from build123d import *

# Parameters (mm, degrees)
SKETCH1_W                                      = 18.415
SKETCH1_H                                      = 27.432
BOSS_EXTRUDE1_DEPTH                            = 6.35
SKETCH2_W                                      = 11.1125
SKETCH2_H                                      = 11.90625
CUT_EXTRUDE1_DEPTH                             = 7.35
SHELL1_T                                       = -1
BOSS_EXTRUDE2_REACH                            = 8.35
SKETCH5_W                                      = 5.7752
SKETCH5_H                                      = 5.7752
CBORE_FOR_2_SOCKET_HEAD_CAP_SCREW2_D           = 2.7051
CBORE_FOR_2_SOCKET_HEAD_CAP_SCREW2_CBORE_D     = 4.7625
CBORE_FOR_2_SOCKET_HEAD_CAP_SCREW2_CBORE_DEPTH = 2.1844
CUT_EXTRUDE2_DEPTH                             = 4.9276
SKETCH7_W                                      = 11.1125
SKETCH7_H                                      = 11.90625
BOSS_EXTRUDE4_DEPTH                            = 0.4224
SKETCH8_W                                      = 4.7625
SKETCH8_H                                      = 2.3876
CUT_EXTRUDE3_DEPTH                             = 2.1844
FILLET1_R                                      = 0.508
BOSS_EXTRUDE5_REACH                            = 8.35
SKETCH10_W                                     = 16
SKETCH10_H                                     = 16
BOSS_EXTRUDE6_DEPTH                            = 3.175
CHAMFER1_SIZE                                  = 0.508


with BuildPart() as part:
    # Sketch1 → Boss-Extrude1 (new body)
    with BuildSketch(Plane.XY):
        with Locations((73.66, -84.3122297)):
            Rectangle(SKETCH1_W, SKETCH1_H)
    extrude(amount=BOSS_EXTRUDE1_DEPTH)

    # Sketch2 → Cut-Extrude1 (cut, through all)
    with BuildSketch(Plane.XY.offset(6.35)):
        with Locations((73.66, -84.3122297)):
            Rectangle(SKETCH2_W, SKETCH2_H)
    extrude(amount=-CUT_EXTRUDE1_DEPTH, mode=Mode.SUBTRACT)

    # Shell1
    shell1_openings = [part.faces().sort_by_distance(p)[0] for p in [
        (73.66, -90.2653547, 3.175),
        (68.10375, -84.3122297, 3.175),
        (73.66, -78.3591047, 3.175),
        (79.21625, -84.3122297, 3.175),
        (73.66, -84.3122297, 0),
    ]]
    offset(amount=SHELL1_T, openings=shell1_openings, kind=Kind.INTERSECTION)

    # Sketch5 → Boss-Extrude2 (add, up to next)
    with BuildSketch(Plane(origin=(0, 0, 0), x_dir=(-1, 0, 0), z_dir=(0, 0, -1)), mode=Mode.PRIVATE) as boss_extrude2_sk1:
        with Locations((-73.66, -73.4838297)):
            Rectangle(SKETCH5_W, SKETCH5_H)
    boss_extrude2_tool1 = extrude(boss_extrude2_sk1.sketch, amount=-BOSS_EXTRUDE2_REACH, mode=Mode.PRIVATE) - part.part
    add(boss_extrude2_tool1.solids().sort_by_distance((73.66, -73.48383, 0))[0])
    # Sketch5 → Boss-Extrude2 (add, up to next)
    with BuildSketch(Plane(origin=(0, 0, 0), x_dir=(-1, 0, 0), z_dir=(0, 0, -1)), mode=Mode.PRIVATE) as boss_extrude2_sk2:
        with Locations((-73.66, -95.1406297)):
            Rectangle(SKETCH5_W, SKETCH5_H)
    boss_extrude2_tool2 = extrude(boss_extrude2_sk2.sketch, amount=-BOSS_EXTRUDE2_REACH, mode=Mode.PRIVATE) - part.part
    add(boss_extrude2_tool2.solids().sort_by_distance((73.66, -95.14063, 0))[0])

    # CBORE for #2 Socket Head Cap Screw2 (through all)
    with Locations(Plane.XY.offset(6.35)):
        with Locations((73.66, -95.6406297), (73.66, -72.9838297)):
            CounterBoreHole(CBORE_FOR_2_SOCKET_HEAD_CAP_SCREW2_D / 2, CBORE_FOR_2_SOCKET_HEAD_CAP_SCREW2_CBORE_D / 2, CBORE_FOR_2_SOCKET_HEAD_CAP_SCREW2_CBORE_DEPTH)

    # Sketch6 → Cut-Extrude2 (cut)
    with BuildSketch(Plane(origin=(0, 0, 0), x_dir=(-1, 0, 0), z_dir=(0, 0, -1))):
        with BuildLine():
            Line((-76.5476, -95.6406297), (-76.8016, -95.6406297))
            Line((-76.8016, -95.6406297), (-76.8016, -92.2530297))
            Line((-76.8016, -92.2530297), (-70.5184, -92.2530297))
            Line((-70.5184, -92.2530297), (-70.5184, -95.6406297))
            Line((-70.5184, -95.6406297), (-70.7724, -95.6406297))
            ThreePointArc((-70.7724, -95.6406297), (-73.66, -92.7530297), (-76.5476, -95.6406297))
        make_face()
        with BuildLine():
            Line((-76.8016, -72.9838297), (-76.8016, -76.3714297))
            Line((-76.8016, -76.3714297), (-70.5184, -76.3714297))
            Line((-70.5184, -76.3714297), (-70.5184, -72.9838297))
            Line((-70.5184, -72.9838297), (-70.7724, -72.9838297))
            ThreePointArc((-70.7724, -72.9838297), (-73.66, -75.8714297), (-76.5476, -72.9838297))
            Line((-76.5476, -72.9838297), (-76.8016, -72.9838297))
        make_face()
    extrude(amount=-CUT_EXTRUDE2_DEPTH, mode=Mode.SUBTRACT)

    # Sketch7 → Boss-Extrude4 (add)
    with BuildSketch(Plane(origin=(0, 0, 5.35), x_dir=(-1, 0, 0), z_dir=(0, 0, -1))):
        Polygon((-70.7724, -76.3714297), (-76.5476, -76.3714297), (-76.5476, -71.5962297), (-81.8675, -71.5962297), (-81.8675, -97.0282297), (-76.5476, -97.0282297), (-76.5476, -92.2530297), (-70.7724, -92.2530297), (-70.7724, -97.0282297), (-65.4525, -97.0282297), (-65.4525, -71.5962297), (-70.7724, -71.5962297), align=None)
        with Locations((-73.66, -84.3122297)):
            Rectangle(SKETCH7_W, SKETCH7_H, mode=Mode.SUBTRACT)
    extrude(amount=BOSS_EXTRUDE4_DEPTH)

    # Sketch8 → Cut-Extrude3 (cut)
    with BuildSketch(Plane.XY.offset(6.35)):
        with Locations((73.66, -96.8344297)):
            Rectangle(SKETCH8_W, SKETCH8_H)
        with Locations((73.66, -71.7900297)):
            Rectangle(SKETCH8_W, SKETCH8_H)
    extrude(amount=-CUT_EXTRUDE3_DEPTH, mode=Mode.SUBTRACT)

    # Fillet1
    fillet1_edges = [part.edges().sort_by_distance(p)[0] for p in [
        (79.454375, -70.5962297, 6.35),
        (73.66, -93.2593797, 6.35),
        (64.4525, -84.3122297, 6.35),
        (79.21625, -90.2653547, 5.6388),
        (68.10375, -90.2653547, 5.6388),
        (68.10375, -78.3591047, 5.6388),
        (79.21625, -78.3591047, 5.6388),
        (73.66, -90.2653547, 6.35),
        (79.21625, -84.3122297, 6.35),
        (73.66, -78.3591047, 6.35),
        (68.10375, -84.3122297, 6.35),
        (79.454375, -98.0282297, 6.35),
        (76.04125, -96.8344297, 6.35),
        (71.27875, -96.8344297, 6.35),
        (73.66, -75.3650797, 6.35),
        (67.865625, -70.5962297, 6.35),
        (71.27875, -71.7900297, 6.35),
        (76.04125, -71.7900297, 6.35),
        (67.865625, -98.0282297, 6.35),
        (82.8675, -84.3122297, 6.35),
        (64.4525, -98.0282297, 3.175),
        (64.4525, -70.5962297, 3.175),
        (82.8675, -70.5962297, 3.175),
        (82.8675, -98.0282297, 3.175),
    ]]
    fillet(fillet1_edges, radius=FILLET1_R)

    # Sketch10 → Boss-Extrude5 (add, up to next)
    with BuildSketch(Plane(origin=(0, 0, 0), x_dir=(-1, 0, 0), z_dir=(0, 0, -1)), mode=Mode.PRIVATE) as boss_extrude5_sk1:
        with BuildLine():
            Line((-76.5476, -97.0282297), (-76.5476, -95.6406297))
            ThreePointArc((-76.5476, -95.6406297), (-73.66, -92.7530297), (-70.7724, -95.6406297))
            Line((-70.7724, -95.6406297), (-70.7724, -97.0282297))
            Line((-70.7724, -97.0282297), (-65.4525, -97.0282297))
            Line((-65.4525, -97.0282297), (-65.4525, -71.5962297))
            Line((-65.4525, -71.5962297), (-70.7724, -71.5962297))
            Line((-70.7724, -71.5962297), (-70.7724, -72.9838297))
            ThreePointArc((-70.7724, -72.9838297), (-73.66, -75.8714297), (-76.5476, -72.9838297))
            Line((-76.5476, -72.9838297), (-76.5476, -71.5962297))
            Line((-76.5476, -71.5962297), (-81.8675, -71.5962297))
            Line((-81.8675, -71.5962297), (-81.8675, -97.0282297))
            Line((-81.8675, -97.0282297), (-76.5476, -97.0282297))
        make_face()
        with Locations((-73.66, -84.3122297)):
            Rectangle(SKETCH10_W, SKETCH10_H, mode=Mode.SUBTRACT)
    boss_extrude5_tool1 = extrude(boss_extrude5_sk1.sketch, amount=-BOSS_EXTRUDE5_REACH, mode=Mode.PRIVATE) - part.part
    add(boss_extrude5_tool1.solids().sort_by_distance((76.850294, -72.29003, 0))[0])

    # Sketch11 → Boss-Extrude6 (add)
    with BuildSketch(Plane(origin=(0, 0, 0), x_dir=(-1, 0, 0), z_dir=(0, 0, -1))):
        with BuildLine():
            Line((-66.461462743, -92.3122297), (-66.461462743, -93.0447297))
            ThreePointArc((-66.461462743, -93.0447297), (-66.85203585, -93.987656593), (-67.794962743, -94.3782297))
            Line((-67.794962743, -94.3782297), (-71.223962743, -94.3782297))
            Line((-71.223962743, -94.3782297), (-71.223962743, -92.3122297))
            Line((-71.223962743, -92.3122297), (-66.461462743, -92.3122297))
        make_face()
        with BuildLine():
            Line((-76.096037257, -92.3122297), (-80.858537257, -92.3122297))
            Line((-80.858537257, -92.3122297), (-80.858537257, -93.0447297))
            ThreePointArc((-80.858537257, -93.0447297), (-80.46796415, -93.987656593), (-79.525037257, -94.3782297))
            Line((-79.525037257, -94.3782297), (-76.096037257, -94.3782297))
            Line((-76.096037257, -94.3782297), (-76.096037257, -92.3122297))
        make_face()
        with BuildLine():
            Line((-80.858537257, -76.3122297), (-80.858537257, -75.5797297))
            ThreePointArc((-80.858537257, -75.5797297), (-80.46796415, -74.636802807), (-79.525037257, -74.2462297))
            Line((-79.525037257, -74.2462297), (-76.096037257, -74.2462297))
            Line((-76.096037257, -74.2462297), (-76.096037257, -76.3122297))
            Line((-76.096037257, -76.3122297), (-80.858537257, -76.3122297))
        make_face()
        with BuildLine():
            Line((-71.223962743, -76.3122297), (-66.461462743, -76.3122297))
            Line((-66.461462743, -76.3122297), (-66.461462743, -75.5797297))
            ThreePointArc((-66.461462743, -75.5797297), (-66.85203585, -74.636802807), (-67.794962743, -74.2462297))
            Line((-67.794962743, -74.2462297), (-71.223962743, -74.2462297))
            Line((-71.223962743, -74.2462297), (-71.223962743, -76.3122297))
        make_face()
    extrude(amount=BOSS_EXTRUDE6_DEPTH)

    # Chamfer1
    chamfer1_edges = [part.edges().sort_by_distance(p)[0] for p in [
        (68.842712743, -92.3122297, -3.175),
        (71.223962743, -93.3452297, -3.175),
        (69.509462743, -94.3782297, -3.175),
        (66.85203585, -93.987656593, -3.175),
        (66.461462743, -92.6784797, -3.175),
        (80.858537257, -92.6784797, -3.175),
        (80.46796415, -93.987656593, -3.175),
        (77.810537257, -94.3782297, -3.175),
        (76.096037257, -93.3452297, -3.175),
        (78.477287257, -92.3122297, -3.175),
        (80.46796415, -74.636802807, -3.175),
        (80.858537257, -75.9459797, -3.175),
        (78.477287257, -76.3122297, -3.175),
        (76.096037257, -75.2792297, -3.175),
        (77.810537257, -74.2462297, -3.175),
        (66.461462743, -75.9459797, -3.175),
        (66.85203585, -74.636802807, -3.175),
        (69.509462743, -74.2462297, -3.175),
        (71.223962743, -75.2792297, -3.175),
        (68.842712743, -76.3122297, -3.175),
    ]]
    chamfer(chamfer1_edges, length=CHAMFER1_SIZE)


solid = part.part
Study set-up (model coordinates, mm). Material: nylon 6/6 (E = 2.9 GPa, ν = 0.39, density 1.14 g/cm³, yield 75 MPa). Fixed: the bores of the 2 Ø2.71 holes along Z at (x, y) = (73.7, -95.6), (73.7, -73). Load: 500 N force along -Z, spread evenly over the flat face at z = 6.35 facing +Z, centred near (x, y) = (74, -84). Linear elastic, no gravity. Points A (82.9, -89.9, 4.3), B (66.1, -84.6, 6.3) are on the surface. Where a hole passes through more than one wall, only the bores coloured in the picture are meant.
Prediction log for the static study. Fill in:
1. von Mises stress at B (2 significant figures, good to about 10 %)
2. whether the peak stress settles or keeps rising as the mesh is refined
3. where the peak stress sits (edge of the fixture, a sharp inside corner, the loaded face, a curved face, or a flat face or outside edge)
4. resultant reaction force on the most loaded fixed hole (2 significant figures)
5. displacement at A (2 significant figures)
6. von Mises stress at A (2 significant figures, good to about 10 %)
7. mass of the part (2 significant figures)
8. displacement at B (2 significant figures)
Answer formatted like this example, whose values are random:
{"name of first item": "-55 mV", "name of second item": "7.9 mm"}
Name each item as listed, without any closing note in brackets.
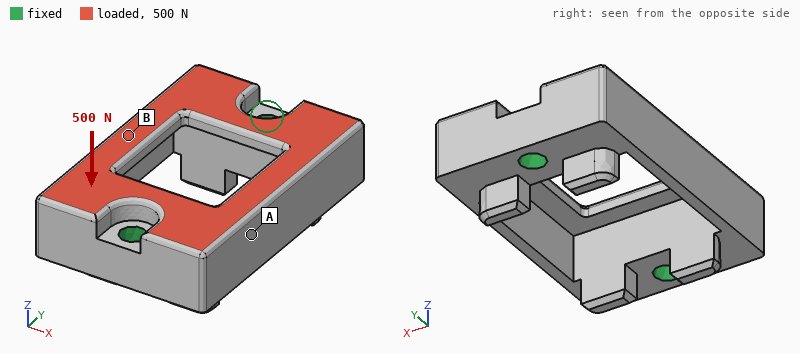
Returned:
{"von Mises stress at B": "16 MPa", "whether the peak stress settles or keeps rising as the mesh is refined": "keeps rising", "where the peak stress sits": "edge of the fixture", "resultant reaction force on the most loaded fixed hole": "260 N", "displacement at A": "0.13 mm", "von Mises stress at A": "3.9 MPa", "mass of the part": "2.0 g", "displacement at B": "0.17 mm"}
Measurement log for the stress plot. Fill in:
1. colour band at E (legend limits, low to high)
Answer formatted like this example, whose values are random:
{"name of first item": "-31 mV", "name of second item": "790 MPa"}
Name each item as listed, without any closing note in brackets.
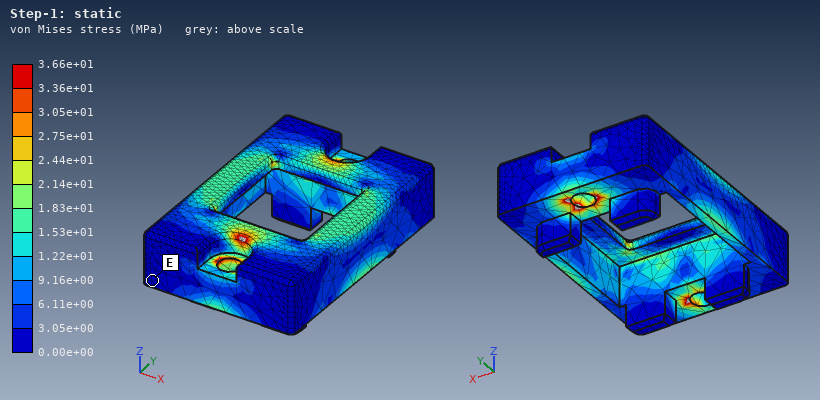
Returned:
{"colour band at E": "0.00e+00 to 3.05e+00 MPa"}
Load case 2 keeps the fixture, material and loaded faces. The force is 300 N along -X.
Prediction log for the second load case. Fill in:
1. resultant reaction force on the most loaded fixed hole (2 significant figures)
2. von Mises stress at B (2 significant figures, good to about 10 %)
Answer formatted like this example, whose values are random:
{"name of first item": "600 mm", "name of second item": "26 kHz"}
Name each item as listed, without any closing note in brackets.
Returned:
{"resultant reaction force on the most loaded fixed hole": "150 N", "von Mises stress at B": "4.2 MPa"}
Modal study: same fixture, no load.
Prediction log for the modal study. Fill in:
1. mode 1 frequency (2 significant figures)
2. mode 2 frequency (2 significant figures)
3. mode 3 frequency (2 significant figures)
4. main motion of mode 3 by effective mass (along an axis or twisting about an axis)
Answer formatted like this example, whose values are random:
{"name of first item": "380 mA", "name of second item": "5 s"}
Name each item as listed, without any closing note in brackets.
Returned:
{"mode 1 frequency": "7100 Hz", "mode 2 frequency": "8400 Hz", "mode 3 frequency": "8700 Hz", "main motion of mode 3 by effective mass": "along Z"}
